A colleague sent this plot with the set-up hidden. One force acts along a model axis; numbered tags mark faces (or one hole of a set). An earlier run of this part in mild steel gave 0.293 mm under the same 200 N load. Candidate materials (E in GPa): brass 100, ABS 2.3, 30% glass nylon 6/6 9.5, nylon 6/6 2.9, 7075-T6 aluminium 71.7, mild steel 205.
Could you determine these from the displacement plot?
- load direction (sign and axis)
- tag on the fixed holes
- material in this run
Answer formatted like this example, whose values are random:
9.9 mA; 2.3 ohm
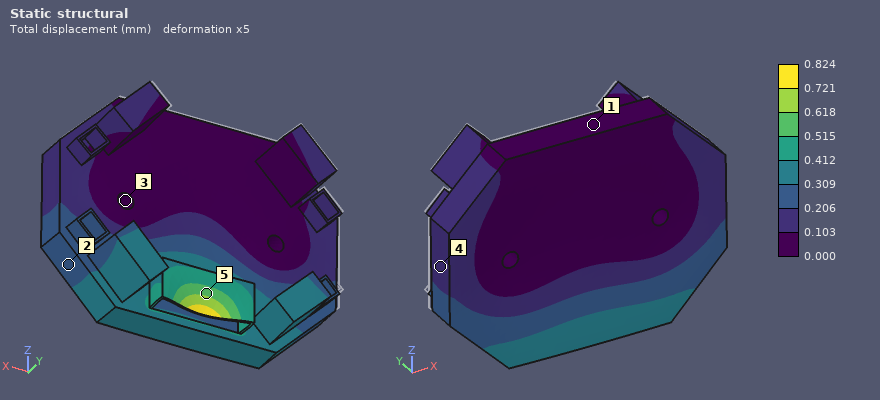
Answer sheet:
-Y; 3; 7075-T6 aluminium
